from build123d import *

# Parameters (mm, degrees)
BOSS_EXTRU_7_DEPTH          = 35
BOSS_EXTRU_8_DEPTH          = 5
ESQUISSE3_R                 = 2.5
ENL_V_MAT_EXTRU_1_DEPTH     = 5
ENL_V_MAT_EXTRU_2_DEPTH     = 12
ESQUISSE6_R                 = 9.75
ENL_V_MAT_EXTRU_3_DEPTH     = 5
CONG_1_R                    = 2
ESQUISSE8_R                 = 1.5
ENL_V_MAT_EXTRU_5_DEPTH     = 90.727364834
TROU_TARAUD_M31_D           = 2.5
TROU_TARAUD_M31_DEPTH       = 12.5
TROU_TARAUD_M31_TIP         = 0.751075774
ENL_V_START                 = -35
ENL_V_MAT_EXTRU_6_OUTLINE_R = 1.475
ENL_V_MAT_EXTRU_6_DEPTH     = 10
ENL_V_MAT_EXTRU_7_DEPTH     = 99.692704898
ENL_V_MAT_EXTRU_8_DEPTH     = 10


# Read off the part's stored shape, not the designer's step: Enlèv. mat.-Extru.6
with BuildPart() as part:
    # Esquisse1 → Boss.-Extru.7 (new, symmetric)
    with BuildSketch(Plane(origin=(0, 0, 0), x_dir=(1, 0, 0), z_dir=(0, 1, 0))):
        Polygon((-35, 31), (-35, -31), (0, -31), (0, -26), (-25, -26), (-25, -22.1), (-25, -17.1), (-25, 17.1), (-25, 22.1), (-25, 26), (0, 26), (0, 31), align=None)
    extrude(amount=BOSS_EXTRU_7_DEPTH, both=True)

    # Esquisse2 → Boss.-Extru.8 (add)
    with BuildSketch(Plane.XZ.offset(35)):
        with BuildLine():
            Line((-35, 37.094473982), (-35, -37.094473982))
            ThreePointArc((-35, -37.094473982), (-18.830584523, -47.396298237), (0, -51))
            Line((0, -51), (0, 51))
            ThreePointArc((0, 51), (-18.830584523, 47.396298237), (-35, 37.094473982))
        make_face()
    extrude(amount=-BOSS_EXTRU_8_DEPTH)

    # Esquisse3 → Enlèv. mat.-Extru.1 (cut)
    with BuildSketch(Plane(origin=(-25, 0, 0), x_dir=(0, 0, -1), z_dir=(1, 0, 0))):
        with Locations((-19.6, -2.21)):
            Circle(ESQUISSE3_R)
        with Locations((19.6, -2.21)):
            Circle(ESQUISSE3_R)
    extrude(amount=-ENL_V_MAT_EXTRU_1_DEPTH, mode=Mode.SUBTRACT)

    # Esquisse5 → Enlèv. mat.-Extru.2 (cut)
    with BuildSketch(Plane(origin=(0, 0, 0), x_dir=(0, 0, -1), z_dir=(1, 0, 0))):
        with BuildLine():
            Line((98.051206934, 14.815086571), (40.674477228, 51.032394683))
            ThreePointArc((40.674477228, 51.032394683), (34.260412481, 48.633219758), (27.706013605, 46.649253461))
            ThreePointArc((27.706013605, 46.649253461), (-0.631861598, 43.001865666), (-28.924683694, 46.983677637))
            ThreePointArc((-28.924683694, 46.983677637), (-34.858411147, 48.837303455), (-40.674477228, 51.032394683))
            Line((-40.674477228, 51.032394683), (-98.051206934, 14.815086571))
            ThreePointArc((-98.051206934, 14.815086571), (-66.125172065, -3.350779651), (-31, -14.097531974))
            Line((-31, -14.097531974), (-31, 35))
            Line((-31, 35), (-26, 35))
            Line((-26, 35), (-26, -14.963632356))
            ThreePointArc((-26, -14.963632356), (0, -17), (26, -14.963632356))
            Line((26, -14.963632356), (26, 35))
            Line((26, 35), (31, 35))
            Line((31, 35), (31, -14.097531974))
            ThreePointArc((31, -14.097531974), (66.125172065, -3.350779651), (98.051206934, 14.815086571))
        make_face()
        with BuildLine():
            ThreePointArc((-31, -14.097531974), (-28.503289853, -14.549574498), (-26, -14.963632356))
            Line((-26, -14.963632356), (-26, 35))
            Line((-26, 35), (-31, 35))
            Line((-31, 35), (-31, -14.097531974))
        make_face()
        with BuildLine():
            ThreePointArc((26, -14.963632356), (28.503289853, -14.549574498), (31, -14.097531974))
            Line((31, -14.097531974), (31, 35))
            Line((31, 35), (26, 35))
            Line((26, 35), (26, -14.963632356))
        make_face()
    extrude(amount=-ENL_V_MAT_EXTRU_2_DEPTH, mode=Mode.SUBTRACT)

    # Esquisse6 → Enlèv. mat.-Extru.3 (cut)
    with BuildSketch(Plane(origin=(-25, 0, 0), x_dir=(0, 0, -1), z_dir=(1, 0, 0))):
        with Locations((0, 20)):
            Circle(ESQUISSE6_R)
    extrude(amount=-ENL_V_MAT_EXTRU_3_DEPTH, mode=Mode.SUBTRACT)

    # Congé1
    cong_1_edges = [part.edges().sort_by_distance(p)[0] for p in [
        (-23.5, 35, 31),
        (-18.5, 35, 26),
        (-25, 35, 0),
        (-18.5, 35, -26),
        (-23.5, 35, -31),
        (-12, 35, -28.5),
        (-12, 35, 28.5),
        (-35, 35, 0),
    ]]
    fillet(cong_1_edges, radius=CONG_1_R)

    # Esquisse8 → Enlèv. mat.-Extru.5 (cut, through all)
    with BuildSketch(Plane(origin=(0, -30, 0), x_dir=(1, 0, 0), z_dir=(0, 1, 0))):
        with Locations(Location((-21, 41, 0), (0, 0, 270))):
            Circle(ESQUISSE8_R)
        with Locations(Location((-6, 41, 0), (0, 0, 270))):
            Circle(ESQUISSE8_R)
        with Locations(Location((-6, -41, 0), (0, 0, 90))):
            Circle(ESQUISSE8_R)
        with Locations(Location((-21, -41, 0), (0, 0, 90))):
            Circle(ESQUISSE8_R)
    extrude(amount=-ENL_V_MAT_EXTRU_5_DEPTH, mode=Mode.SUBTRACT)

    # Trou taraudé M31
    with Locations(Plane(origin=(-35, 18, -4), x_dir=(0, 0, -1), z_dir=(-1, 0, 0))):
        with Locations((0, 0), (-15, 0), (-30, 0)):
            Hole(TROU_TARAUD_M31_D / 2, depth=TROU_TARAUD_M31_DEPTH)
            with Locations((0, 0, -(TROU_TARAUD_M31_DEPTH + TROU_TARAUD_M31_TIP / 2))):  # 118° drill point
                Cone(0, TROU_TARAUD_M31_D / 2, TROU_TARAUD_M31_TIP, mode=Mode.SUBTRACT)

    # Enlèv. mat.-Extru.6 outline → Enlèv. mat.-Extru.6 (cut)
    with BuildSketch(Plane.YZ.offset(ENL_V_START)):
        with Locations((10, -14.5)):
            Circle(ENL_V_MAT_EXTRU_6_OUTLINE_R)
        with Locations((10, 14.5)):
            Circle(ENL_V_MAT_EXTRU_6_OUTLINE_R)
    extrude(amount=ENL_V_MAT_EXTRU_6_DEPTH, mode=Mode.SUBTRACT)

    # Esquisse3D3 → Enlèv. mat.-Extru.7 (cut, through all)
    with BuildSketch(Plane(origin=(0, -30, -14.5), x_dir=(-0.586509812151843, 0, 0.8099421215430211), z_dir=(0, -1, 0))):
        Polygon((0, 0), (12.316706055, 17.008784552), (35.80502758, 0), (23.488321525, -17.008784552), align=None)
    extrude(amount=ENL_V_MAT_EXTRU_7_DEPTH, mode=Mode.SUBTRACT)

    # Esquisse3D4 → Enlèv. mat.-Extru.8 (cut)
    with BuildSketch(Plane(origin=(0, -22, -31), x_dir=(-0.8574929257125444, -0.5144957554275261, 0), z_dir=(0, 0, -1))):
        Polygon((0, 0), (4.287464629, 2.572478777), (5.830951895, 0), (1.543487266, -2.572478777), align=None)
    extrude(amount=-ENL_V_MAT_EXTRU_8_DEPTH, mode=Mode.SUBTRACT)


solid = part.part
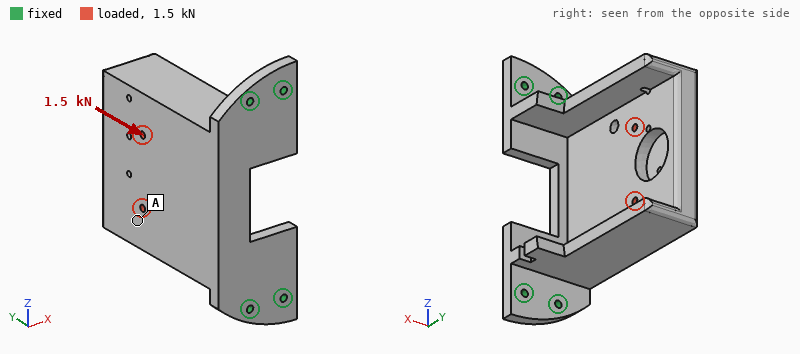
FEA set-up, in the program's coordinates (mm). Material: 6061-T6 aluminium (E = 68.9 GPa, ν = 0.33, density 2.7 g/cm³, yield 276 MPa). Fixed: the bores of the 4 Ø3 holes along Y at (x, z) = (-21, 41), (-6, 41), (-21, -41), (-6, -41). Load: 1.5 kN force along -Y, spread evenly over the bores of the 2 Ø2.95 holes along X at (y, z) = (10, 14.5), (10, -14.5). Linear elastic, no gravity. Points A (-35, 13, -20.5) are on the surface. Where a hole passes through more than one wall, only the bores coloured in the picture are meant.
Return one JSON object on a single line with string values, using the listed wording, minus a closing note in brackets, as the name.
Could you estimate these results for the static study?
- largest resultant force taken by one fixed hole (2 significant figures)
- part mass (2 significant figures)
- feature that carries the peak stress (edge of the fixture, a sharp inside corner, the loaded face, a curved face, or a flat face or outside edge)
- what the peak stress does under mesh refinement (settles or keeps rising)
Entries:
{"largest resultant force taken by one fixed hole": "1.1 kN", "part mass": "170 g", "feature that carries the peak stress": "edge of the fixture", "what the peak stress does under mesh refinement": "keeps rising"}
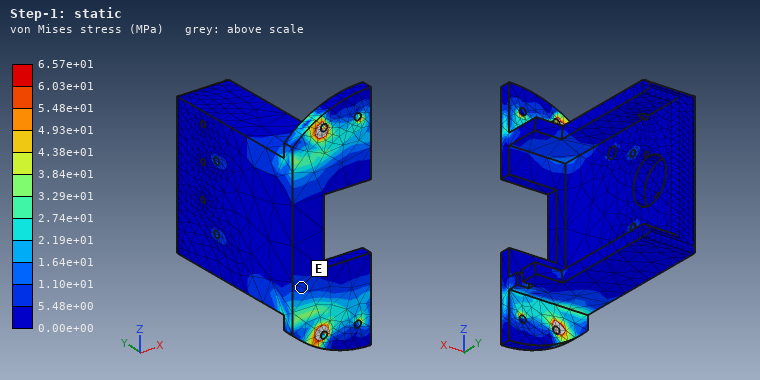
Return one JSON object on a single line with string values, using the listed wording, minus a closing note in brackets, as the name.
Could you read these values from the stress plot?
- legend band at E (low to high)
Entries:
{"legend band at E": "5.48e+00 to 1.10e+01 MPa"}
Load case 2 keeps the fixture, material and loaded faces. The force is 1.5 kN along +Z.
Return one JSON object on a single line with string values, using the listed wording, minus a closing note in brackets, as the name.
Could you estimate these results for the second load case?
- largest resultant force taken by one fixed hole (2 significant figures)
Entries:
{"largest resultant force taken by one fixed hole": "980 N"}
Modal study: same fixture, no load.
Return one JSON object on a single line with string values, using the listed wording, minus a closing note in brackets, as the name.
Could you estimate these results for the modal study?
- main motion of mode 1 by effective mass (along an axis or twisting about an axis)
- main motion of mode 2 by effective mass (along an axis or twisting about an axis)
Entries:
{"main motion of mode 1 by effective mass": "along X", "main motion of mode 2 by effective mass": "along Z"}
